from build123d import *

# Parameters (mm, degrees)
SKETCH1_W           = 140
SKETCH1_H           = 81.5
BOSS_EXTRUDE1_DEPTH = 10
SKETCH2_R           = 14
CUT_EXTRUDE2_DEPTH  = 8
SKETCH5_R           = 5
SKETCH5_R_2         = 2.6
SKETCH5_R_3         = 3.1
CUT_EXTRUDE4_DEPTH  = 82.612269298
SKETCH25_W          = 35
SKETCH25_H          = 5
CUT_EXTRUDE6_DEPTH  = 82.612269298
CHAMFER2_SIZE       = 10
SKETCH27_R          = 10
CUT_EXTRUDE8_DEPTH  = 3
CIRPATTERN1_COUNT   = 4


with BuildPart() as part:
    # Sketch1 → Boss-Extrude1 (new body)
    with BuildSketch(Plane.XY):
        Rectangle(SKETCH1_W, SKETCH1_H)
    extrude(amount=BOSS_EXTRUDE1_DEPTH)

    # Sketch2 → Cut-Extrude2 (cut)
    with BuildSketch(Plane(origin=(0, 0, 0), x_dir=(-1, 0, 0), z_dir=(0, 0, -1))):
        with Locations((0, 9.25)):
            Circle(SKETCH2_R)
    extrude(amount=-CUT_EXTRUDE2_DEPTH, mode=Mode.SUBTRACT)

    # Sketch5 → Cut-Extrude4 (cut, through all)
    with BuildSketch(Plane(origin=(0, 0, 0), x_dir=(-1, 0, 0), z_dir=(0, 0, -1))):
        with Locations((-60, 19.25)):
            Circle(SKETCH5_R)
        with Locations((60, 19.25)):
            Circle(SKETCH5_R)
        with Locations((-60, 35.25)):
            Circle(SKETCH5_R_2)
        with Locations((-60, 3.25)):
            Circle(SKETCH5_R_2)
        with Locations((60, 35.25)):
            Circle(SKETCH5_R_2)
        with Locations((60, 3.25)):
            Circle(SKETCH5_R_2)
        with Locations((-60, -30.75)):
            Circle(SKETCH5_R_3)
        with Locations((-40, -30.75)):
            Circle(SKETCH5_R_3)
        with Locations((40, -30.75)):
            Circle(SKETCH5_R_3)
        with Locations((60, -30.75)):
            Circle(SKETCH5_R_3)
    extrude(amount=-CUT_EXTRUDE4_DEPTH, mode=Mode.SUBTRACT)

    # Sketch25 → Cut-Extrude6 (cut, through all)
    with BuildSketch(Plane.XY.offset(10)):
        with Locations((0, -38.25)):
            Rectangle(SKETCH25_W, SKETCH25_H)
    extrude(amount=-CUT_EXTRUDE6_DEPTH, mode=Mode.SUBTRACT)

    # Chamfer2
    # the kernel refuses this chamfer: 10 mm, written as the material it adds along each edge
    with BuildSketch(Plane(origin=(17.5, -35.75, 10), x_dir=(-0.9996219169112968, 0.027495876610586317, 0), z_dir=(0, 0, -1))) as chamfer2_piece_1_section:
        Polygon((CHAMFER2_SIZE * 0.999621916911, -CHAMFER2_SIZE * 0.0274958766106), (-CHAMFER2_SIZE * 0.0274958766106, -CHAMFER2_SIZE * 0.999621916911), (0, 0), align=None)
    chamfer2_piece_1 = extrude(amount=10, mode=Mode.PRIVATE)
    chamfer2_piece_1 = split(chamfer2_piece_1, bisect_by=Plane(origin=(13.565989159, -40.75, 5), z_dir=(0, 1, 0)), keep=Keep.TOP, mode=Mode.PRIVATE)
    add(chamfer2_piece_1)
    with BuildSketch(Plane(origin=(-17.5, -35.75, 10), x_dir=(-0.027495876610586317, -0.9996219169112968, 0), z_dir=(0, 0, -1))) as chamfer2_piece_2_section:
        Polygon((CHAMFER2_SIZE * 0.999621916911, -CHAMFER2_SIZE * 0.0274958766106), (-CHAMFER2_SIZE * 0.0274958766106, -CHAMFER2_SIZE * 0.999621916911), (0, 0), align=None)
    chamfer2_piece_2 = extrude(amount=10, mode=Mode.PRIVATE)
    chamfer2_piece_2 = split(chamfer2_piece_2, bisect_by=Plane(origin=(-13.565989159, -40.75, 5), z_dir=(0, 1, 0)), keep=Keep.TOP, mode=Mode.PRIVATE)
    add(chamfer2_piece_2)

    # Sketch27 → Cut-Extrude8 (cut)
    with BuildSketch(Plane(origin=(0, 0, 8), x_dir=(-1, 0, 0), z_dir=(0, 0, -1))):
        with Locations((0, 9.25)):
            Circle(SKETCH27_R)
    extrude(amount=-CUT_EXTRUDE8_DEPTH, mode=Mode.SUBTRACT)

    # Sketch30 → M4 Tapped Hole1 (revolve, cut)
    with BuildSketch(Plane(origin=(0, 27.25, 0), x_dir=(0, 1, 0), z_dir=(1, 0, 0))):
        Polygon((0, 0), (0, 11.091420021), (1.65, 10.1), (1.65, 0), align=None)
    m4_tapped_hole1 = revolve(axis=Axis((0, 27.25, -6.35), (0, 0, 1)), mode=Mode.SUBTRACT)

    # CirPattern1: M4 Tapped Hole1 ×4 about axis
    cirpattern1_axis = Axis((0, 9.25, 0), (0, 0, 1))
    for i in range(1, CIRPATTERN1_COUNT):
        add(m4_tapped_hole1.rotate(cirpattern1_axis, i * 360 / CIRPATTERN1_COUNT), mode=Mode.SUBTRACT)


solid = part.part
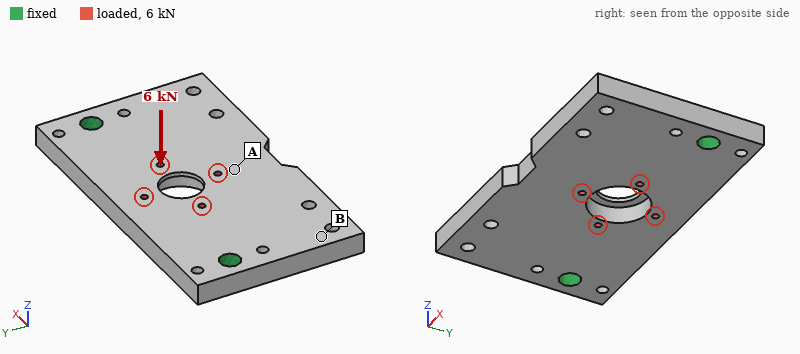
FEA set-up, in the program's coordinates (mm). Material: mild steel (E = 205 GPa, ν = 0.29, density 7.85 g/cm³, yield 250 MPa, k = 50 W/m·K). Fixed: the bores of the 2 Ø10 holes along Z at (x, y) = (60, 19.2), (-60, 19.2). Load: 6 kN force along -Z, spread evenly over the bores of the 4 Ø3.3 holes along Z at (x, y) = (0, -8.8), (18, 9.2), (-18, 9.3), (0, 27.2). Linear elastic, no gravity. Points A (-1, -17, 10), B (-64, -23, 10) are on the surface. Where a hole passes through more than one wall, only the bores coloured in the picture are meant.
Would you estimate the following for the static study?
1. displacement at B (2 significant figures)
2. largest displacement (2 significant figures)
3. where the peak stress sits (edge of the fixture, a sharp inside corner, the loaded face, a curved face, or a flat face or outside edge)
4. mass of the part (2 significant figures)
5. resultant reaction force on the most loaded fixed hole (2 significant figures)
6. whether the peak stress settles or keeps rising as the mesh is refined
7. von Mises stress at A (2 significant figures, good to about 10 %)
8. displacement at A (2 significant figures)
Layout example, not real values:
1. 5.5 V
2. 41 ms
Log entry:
1. 17 µm
2. 86 µm
3. edge of the fixture
4. 810 g
5. 3.0 kN
6. keeps rising
7. 71 MPa
8. 78 µm
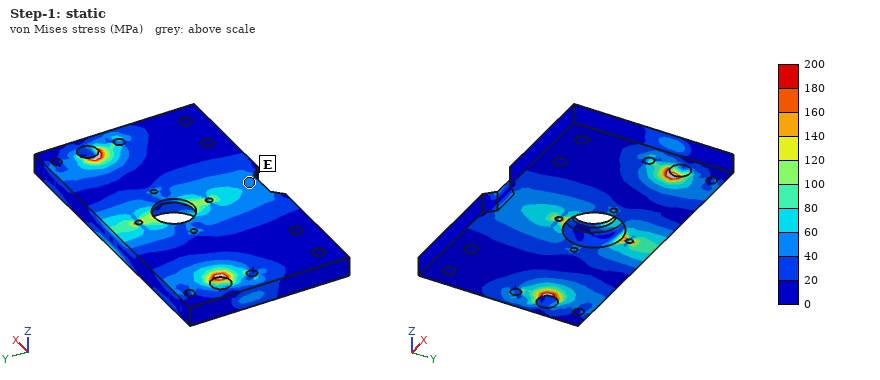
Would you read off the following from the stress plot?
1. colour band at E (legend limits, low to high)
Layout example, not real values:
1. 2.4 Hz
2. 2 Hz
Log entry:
1. 40 to 60 MPa
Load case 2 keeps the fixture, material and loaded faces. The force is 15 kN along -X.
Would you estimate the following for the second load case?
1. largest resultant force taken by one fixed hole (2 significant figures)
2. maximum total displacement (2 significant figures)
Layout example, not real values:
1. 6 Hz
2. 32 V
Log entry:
1. 7.6 kN
2. 6.5 µm
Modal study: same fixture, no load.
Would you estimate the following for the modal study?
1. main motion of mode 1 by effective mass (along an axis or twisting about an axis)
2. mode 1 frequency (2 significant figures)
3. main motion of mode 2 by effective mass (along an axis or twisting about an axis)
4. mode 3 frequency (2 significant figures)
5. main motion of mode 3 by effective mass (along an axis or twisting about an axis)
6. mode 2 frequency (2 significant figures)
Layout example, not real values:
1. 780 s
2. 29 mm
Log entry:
1. along Z
2. 1600 Hz
3. twisting about Y
4. 3600 Hz
5. along Z
6. 3100 Hz
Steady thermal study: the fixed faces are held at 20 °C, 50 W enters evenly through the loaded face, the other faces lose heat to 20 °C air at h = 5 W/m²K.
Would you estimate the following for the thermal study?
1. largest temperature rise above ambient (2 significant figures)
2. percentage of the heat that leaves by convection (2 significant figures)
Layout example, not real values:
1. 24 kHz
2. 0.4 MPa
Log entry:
1. 51 K
2. 7.1 %
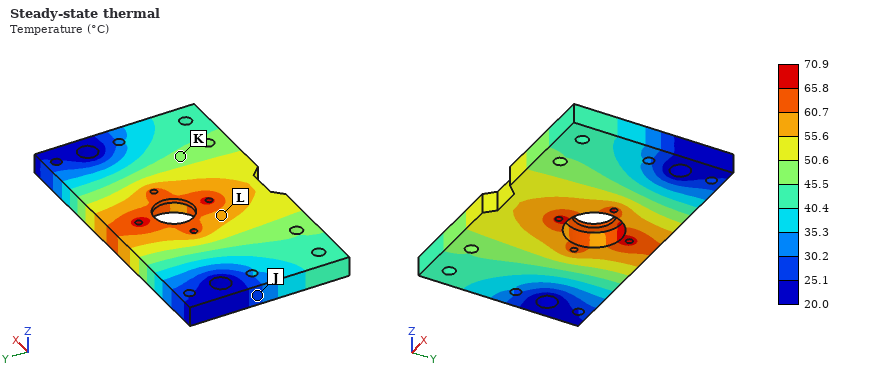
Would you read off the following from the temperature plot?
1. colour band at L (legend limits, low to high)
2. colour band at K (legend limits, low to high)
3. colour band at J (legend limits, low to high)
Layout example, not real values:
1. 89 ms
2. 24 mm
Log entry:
1. 55.6 to 60.7 °C
2. 45.5 to 50.6 °C
3. 25.1 to 30.2 °C
